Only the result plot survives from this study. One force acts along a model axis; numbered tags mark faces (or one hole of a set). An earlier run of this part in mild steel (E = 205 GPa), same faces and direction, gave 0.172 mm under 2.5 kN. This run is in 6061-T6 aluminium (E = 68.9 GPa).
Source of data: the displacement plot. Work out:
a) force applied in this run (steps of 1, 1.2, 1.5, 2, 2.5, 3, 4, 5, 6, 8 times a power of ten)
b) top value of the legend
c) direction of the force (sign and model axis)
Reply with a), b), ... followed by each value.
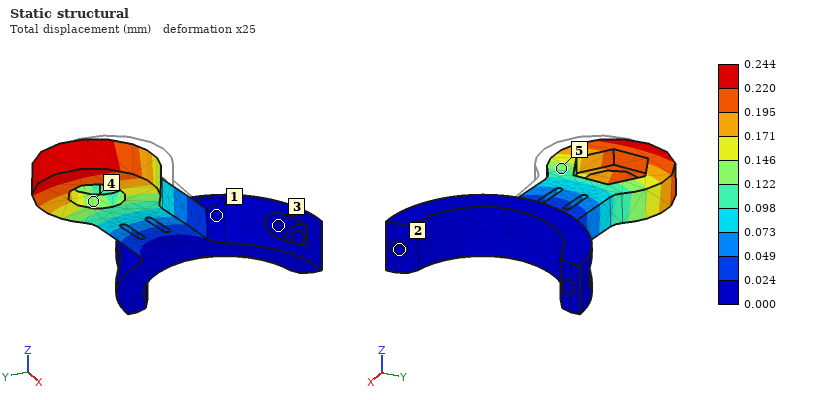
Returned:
a) 1.2 kN
b) 0.244 mm
c) +Y
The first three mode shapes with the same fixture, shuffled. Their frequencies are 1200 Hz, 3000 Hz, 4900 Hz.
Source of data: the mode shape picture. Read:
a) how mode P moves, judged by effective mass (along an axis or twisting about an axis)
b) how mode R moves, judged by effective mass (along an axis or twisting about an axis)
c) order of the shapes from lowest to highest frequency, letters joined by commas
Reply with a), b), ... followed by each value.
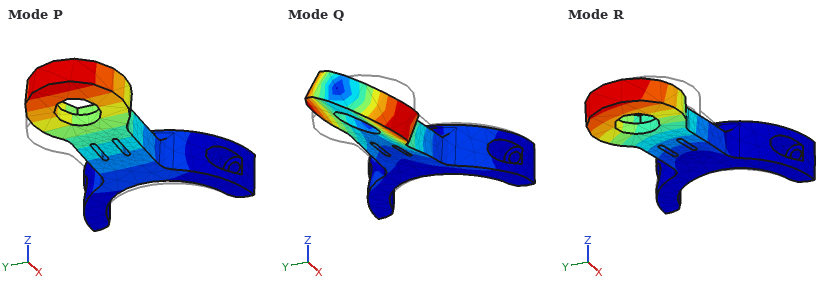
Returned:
a) along Z
b) along Y
c) P, R, Q
